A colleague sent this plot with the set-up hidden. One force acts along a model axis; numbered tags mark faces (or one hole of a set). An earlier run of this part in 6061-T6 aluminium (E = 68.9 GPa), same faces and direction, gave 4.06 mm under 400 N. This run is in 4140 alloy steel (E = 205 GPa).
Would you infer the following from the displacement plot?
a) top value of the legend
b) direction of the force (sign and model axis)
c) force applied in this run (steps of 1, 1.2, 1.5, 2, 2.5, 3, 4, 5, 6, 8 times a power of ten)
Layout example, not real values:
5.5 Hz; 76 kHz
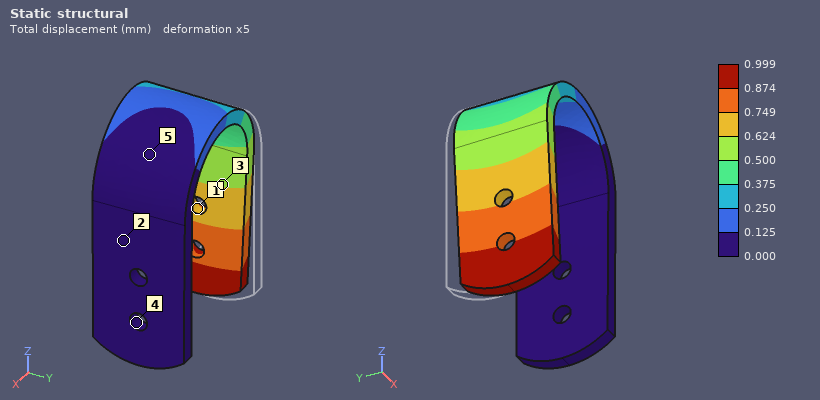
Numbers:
0.999 mm; -Y; 300 N
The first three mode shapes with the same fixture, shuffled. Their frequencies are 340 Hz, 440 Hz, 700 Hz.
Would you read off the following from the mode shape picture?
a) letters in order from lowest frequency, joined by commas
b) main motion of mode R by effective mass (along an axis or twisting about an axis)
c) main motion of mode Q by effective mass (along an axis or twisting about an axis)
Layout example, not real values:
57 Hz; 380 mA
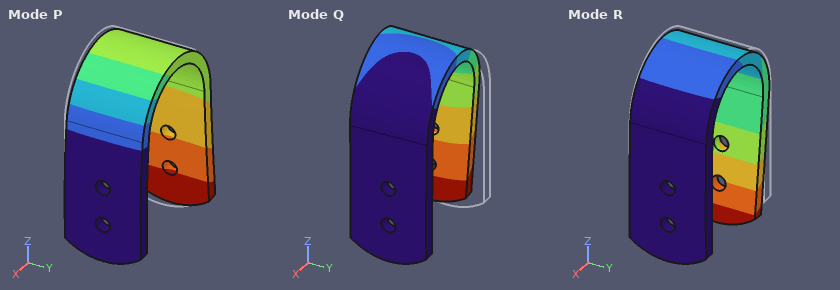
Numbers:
R, Q, P; along Z; along Y
